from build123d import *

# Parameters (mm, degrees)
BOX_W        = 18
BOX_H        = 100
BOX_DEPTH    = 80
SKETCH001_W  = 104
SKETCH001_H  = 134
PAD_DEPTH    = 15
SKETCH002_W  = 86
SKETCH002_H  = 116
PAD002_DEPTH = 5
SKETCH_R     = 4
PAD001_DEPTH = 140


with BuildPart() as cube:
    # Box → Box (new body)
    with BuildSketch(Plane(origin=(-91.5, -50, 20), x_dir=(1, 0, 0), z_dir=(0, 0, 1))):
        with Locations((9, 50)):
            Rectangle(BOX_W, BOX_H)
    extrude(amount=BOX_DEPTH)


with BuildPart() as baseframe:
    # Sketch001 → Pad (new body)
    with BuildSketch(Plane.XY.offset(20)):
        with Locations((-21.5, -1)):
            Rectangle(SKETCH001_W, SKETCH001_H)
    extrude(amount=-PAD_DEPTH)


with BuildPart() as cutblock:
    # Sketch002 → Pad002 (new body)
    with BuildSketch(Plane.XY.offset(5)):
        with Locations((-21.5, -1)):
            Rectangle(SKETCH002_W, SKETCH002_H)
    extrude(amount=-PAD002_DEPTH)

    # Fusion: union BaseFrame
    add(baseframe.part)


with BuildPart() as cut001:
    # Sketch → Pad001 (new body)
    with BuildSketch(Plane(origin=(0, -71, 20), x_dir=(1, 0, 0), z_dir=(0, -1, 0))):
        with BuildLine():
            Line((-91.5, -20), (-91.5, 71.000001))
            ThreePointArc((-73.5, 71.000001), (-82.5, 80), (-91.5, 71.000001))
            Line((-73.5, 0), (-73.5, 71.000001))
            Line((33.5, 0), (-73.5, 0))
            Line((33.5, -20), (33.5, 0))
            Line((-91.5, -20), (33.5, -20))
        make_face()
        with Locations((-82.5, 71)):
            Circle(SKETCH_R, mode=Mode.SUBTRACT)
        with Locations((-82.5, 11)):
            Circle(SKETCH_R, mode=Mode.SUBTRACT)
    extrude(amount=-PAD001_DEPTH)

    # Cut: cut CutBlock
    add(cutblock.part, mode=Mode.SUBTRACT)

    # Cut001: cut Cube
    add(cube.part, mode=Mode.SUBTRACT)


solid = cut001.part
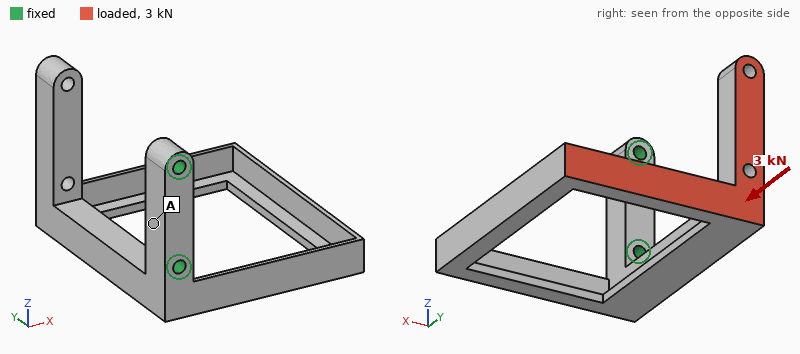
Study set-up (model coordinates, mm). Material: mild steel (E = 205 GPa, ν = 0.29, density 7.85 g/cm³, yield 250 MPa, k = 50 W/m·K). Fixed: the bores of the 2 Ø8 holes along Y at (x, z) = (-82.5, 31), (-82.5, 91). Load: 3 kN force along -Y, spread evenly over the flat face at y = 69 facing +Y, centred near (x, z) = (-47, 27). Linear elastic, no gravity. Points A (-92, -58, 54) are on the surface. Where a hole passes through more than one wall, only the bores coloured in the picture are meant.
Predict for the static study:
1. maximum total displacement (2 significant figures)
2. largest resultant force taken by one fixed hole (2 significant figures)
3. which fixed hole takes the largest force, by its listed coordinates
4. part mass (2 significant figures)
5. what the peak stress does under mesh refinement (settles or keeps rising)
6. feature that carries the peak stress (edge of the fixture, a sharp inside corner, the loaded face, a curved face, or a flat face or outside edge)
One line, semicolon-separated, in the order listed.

0.75 mm; 3.0 kN; (-82.5, 31); 1.1 kg; keeps rising; edge of the fixture
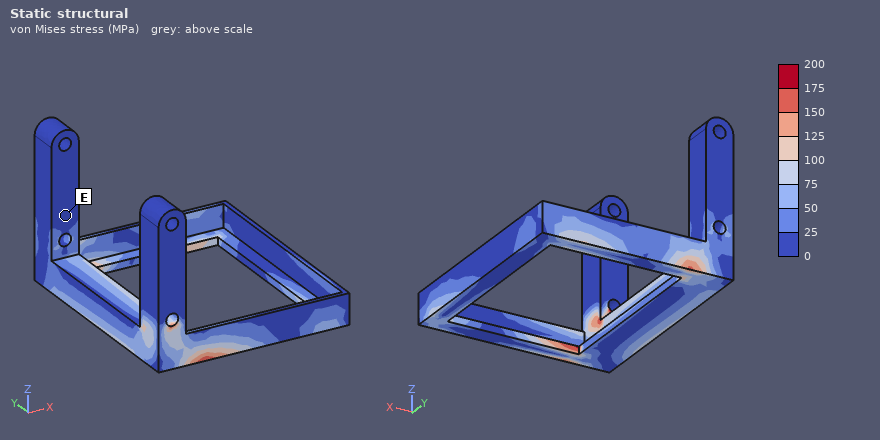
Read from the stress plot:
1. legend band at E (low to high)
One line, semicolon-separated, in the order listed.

0 to 25 MPa
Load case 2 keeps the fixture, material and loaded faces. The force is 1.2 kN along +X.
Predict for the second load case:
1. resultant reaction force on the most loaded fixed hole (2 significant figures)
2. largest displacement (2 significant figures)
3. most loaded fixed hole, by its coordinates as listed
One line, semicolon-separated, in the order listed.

1.2 kN; 0.58 mm; (-82.5, 31)
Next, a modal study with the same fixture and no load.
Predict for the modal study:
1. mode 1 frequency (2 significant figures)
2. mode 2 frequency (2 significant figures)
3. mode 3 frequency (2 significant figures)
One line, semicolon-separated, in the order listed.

340 Hz; 360 Hz; 530 Hz
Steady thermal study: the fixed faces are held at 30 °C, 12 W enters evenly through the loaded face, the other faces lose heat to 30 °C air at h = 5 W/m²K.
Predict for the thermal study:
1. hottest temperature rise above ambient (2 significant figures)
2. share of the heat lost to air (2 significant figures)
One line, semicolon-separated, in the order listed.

61 K; 46 %
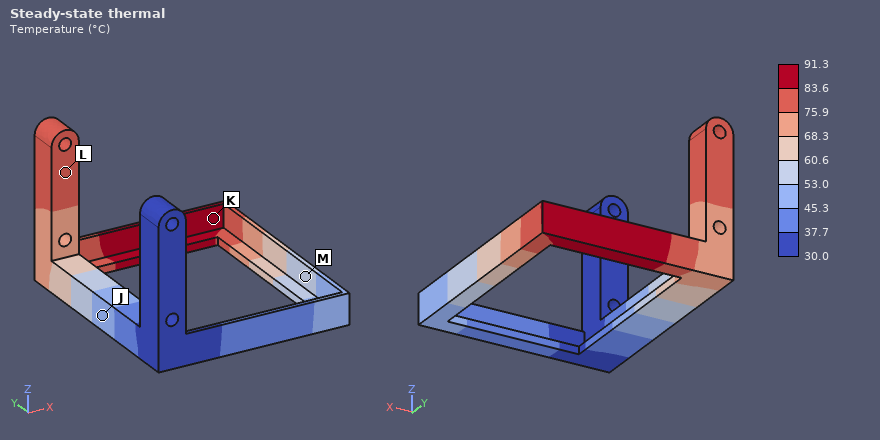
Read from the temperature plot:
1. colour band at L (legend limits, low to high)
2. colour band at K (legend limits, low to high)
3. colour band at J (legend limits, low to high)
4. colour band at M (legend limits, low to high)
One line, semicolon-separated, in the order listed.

75.9 to 83.6 °C; 83.6 to 91.3 °C; 45.3 to 53.0 °C; 53.0 to 60.6 °C
